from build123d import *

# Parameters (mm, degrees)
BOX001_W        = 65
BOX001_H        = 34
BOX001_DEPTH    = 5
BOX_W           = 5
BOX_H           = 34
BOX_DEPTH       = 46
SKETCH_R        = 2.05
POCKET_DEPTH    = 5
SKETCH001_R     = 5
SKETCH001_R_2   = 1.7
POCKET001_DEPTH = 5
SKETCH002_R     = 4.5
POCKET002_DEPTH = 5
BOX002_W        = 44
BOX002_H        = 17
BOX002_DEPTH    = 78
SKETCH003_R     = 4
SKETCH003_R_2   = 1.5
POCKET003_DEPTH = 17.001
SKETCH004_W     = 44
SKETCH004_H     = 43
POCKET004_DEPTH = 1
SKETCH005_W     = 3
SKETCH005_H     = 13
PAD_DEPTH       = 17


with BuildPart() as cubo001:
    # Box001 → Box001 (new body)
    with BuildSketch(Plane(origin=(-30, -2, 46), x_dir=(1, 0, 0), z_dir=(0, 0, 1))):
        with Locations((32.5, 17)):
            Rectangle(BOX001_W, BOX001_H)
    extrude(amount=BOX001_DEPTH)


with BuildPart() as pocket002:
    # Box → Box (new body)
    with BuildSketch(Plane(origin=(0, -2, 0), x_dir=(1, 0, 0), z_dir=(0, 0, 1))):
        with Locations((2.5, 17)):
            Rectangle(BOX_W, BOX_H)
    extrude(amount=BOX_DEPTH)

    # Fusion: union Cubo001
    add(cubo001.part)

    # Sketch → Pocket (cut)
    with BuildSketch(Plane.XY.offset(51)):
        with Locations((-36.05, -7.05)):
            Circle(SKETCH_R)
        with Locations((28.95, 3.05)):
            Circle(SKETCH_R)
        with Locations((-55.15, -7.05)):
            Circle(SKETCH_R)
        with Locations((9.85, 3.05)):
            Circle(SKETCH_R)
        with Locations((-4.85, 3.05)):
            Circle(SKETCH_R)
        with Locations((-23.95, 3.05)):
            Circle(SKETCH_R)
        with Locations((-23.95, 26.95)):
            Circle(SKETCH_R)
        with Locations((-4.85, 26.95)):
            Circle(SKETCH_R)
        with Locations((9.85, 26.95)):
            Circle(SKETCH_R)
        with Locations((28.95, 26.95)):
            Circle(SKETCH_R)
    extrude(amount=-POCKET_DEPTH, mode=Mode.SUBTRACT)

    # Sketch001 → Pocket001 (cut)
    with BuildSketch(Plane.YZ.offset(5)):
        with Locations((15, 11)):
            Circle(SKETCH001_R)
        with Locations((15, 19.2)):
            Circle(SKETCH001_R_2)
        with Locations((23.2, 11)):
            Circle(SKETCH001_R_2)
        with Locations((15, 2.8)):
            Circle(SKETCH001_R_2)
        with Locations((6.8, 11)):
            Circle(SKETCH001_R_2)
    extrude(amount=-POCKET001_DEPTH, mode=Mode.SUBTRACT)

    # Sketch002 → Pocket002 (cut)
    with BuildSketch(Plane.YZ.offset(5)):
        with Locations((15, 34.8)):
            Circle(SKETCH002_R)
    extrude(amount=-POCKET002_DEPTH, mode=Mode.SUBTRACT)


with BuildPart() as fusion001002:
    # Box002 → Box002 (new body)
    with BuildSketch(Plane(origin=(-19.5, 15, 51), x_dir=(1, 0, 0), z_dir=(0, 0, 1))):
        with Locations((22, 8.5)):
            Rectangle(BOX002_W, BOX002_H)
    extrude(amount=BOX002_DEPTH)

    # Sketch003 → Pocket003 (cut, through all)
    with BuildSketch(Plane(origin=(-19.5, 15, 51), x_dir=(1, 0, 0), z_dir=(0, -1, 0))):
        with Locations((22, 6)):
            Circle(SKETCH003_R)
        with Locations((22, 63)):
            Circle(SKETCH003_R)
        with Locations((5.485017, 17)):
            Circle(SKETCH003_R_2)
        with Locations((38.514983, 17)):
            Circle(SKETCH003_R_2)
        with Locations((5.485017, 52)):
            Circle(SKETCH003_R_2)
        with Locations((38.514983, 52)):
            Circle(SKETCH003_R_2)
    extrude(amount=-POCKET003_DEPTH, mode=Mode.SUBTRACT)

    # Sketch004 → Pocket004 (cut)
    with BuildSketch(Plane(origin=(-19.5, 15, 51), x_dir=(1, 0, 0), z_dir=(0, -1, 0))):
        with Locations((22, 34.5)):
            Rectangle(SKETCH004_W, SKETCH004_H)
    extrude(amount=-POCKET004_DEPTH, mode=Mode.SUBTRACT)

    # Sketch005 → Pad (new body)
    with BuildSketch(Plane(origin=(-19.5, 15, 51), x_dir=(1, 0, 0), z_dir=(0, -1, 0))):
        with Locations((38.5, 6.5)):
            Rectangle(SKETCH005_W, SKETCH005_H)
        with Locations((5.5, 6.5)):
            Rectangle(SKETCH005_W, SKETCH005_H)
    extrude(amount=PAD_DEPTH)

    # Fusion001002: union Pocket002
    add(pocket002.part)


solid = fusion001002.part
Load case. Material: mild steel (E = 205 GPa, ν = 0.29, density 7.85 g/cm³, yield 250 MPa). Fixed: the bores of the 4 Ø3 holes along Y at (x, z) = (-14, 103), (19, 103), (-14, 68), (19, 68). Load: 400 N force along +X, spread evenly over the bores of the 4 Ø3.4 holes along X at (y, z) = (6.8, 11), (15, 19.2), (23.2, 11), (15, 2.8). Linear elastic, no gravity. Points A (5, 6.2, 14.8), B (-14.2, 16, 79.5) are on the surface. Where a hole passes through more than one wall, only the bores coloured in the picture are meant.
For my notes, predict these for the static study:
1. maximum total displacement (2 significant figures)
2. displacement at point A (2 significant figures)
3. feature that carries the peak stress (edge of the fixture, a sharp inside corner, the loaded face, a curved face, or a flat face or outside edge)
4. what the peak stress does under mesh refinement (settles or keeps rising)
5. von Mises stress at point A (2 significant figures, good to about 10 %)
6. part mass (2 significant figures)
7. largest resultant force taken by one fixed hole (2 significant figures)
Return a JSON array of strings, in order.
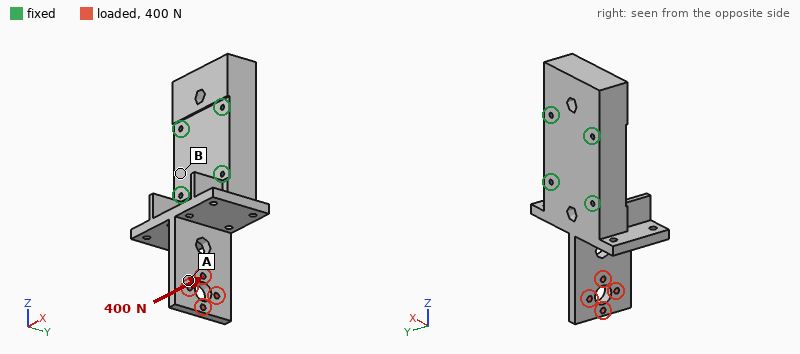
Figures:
["0.16 mm", "0.092 mm", "a sharp inside corner", "keeps rising", "17 MPa", "570 g", "650 N"]
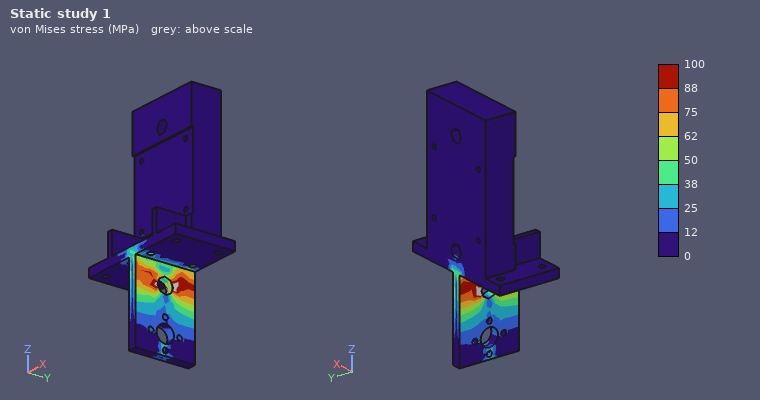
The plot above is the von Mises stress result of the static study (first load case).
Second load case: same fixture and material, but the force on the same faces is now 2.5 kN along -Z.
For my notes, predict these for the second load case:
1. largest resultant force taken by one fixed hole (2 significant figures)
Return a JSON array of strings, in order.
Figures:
["1.1 kN"]
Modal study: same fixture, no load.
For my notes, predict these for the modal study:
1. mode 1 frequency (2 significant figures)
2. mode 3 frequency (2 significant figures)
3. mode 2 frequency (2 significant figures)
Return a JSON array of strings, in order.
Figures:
["1800 Hz", "5000 Hz", "3900 Hz"]
